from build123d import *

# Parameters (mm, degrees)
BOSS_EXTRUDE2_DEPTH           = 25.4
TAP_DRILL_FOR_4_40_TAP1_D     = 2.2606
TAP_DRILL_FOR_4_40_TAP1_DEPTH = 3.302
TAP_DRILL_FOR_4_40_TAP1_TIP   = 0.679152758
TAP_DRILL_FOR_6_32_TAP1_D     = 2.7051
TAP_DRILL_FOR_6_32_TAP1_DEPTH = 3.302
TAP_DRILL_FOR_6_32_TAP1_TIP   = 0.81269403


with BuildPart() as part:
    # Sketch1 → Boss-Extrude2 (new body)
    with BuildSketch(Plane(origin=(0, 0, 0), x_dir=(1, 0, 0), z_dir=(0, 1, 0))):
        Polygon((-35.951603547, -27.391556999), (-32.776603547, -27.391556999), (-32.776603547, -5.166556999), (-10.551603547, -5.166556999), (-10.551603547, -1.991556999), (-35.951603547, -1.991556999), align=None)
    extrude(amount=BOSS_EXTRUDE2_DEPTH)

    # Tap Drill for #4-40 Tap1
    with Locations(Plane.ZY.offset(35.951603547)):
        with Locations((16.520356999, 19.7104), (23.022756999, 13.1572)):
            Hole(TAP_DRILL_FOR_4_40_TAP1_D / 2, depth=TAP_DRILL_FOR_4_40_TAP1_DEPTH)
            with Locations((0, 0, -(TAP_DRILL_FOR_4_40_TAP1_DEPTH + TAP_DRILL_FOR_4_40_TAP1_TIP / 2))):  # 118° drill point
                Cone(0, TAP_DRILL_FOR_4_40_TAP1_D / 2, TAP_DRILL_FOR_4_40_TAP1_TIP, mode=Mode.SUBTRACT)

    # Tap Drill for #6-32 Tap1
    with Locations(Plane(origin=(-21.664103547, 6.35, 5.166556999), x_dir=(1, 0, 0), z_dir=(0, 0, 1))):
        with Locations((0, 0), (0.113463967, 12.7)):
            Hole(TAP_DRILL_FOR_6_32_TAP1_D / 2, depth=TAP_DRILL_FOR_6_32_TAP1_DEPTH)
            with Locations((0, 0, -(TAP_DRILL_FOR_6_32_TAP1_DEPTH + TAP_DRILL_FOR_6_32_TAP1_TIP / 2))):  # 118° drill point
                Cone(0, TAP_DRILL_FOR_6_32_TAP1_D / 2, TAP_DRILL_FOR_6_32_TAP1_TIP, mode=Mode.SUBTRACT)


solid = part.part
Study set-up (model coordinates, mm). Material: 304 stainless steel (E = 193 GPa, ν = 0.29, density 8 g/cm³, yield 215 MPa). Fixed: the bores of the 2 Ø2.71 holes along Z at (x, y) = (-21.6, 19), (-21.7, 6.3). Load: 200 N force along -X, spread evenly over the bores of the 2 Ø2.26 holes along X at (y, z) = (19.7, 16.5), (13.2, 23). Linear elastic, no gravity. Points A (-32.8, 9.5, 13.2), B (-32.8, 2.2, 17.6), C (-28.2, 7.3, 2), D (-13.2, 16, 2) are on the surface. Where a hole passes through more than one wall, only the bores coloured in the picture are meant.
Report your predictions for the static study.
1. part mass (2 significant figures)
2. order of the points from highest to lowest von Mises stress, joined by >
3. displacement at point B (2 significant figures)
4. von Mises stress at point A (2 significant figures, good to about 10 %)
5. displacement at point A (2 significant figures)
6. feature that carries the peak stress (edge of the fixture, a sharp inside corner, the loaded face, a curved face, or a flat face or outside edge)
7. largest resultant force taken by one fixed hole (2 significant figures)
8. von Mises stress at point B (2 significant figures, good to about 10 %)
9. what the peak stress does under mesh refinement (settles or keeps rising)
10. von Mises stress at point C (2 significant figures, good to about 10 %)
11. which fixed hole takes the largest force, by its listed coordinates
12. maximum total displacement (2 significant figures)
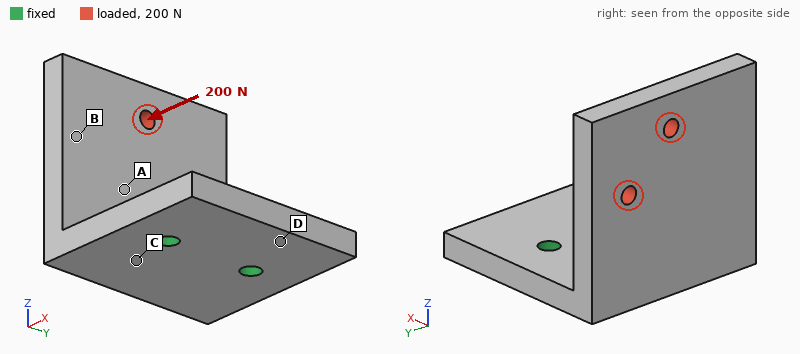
30 g
C > A > B > D
0.053 mm
33 MPa
0.037 mm
edge of the fixture
160 N
20 MPa
keeps rising
64 MPa
(-21.6, 19)
0.11 mm
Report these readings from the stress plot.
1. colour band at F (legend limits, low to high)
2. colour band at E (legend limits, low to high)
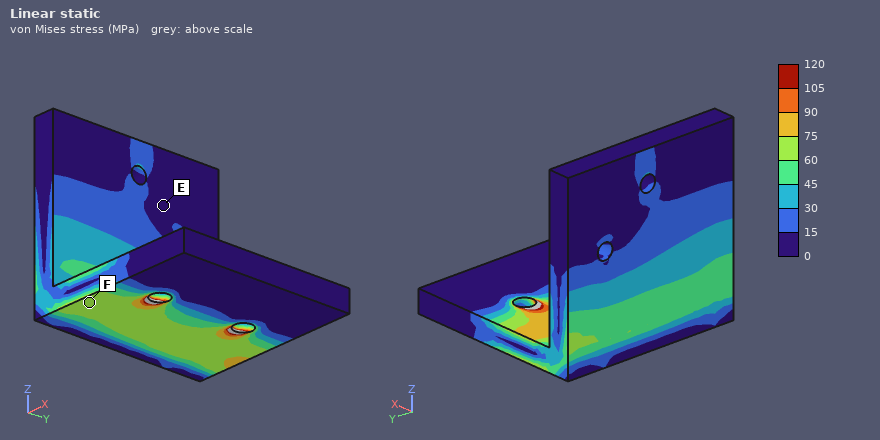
60 to 75 MPa
0 to 15 MPa
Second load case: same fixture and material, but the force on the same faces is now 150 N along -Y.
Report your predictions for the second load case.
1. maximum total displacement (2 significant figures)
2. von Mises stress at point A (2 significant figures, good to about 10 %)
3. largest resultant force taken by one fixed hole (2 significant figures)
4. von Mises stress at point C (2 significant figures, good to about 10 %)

21 µm
8.9 MPa
210 N
23 MPa
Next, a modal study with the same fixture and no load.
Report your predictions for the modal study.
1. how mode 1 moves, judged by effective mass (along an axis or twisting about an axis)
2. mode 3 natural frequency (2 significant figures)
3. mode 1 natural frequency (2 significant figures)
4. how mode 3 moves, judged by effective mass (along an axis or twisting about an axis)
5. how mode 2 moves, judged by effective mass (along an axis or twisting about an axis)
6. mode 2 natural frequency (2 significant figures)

along X
7800 Hz
2400 Hz
along Z
along Y
4500 Hz
